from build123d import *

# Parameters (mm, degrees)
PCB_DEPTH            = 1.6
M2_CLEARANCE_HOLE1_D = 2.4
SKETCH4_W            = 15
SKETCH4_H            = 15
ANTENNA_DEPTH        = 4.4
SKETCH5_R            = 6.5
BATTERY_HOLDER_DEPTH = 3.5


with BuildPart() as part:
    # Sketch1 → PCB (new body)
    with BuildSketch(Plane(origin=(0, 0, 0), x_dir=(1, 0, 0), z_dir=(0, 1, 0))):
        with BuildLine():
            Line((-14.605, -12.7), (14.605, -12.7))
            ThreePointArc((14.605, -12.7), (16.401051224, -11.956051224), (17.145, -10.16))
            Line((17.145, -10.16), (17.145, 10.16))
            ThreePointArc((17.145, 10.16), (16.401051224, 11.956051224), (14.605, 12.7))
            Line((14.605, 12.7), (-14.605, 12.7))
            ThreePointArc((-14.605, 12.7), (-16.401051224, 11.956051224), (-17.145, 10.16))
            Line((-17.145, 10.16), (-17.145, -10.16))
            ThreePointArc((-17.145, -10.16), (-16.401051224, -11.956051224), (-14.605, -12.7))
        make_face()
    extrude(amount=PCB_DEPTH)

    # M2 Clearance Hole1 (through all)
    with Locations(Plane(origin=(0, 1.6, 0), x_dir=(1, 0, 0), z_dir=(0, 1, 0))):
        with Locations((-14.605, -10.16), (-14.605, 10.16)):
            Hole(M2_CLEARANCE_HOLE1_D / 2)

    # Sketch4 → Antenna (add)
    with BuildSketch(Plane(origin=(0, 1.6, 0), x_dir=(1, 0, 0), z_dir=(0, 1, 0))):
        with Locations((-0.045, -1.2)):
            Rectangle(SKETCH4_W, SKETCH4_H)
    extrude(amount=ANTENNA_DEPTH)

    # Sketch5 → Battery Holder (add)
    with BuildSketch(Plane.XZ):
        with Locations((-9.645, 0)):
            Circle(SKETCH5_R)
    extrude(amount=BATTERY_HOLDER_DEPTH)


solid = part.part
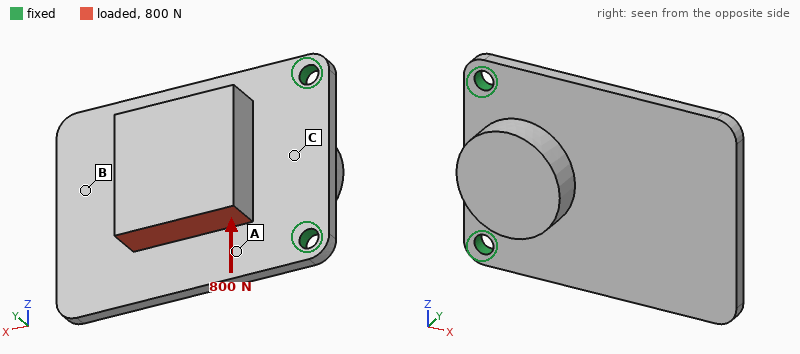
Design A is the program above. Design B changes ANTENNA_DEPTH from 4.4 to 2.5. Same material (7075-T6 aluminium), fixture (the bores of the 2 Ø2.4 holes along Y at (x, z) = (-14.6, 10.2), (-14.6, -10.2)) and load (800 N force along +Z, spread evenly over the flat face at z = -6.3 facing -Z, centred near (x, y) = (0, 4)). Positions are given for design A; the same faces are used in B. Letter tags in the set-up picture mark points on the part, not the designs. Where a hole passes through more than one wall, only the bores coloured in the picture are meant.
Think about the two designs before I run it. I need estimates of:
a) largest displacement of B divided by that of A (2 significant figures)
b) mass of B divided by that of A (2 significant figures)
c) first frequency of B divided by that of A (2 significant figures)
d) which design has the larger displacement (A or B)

0.86
0.85
1.1
A
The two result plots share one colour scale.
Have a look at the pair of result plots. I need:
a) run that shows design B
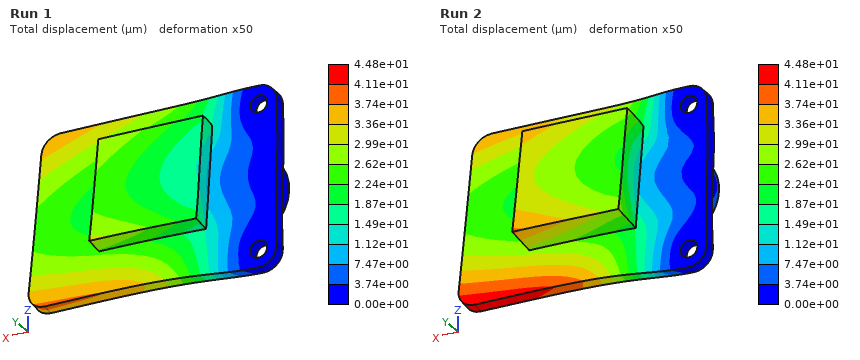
Run 1
